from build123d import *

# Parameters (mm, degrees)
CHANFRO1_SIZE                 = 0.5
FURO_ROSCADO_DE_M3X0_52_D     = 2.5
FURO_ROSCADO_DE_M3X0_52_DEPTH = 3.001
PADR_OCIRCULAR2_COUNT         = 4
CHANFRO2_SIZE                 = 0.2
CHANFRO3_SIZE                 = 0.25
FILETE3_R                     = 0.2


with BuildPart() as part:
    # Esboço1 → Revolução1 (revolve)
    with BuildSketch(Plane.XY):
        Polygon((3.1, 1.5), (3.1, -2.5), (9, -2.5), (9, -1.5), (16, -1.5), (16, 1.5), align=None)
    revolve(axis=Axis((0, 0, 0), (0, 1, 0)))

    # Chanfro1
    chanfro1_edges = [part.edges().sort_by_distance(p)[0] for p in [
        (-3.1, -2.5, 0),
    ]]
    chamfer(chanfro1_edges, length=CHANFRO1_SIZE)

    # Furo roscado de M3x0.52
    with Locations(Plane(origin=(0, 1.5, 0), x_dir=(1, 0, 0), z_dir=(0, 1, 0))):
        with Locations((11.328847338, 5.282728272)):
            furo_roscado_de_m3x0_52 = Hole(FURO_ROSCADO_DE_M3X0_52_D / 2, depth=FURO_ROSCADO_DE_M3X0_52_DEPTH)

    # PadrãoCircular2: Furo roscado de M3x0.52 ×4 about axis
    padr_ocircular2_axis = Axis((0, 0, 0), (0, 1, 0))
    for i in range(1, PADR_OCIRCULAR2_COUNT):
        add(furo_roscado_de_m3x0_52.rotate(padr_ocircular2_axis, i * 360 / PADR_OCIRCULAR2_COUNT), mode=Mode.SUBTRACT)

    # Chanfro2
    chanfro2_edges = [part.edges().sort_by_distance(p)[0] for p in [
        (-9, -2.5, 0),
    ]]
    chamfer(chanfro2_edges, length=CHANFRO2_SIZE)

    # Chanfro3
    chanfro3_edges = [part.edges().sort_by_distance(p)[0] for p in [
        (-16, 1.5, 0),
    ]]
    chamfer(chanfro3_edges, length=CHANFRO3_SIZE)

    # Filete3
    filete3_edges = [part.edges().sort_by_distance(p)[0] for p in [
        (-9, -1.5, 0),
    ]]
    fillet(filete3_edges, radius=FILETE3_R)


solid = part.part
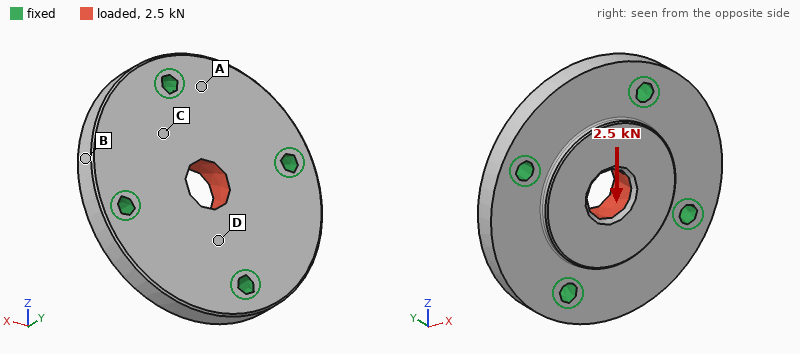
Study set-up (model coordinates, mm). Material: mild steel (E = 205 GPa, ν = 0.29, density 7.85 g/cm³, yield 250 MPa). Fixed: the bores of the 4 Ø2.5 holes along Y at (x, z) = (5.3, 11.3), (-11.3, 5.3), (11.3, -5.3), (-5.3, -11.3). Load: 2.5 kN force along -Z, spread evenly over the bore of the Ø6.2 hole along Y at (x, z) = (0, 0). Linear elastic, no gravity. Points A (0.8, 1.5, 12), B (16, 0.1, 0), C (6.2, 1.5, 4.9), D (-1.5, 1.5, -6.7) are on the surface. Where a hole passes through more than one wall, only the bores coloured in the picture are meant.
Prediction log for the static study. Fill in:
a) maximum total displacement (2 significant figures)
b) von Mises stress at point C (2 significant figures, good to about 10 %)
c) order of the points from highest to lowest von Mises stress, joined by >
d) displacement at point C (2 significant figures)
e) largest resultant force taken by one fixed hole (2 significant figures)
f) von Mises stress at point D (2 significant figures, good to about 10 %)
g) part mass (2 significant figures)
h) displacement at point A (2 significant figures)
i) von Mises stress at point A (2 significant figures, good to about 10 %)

1.8 µm
24 MPa
D > C > A > B
0.71 µm
760 N
35 MPa
19 g
0.72 µm
15 MPa
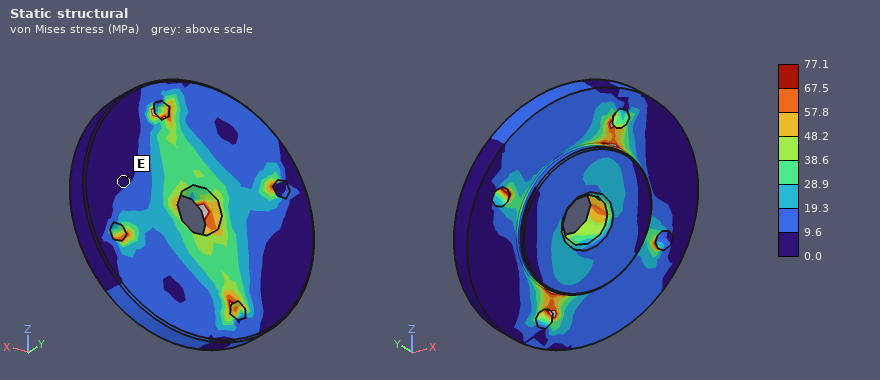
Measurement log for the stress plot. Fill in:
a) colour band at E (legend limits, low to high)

0.0 to 9.6 MPa
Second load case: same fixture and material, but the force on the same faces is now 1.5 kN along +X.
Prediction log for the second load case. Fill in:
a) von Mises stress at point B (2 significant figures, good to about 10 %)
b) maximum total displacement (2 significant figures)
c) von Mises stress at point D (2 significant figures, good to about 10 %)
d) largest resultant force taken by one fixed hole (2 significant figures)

8.1 MPa
1.1 µm
12 MPa
450 N
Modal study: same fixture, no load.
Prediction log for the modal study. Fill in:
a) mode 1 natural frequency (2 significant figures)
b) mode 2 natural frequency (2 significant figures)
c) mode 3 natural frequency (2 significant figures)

35 kHz
36 kHz
37 kHz
